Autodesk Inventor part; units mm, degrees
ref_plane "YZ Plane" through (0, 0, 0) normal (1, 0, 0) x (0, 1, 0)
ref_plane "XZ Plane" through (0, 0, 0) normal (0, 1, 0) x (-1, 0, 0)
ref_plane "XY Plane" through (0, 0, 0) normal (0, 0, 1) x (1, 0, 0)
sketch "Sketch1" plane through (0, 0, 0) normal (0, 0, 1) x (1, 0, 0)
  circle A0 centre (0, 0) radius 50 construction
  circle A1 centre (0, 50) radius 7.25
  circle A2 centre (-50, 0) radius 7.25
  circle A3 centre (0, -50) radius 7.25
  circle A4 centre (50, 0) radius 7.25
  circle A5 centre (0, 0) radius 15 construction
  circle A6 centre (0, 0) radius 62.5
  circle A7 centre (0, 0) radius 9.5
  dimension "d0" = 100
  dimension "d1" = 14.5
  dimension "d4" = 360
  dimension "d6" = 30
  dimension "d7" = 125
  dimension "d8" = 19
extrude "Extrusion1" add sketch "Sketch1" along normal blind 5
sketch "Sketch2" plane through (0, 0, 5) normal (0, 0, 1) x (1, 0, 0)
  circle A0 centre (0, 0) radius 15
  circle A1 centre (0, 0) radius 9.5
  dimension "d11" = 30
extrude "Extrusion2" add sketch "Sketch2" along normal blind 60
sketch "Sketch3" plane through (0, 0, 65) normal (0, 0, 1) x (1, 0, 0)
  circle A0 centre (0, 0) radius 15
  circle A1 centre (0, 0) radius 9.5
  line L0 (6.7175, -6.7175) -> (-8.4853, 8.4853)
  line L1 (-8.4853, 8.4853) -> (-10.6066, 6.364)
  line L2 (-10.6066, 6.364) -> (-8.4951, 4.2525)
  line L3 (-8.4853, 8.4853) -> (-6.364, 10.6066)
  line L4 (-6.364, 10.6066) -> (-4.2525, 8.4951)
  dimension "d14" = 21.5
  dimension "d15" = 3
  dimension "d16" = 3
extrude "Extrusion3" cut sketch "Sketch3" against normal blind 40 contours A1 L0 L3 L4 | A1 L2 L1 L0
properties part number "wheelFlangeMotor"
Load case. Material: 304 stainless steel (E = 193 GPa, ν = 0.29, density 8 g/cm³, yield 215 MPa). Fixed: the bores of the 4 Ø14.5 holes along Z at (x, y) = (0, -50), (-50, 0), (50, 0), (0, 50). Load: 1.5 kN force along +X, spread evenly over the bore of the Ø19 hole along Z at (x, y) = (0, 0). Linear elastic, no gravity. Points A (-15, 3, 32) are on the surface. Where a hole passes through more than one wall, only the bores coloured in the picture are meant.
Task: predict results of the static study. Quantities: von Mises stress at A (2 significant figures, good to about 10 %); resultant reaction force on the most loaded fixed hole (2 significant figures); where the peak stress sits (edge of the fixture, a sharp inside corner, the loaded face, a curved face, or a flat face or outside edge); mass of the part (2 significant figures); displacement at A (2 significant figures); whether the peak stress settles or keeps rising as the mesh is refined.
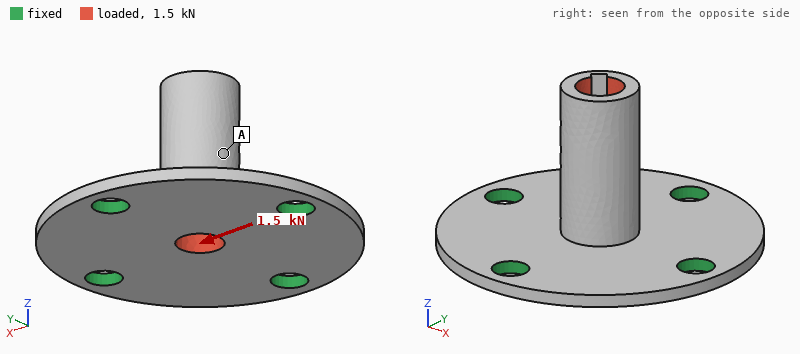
5.3 MPa
790 N
edge of the fixture
650 g
35 µm
keeps rising
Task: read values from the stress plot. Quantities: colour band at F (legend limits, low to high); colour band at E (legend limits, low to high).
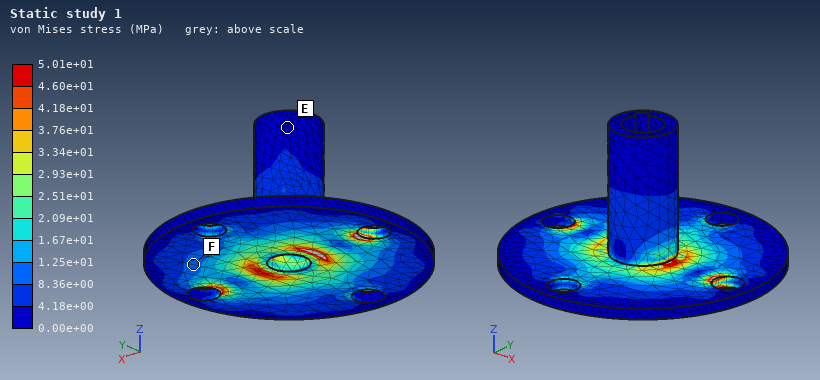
8.36e+00 to 1.25e+01 MPa
0.00e+00 to 4.18e+00 MPa
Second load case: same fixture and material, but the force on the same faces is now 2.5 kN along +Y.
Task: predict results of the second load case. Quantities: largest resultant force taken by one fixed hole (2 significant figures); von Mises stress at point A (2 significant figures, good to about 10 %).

1.3 kN
9.5 MPa
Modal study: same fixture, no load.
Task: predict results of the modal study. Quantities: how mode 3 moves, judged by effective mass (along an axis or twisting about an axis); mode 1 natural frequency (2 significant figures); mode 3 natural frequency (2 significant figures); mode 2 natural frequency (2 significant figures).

along Z
1900 Hz
2900 Hz
1900 Hz
